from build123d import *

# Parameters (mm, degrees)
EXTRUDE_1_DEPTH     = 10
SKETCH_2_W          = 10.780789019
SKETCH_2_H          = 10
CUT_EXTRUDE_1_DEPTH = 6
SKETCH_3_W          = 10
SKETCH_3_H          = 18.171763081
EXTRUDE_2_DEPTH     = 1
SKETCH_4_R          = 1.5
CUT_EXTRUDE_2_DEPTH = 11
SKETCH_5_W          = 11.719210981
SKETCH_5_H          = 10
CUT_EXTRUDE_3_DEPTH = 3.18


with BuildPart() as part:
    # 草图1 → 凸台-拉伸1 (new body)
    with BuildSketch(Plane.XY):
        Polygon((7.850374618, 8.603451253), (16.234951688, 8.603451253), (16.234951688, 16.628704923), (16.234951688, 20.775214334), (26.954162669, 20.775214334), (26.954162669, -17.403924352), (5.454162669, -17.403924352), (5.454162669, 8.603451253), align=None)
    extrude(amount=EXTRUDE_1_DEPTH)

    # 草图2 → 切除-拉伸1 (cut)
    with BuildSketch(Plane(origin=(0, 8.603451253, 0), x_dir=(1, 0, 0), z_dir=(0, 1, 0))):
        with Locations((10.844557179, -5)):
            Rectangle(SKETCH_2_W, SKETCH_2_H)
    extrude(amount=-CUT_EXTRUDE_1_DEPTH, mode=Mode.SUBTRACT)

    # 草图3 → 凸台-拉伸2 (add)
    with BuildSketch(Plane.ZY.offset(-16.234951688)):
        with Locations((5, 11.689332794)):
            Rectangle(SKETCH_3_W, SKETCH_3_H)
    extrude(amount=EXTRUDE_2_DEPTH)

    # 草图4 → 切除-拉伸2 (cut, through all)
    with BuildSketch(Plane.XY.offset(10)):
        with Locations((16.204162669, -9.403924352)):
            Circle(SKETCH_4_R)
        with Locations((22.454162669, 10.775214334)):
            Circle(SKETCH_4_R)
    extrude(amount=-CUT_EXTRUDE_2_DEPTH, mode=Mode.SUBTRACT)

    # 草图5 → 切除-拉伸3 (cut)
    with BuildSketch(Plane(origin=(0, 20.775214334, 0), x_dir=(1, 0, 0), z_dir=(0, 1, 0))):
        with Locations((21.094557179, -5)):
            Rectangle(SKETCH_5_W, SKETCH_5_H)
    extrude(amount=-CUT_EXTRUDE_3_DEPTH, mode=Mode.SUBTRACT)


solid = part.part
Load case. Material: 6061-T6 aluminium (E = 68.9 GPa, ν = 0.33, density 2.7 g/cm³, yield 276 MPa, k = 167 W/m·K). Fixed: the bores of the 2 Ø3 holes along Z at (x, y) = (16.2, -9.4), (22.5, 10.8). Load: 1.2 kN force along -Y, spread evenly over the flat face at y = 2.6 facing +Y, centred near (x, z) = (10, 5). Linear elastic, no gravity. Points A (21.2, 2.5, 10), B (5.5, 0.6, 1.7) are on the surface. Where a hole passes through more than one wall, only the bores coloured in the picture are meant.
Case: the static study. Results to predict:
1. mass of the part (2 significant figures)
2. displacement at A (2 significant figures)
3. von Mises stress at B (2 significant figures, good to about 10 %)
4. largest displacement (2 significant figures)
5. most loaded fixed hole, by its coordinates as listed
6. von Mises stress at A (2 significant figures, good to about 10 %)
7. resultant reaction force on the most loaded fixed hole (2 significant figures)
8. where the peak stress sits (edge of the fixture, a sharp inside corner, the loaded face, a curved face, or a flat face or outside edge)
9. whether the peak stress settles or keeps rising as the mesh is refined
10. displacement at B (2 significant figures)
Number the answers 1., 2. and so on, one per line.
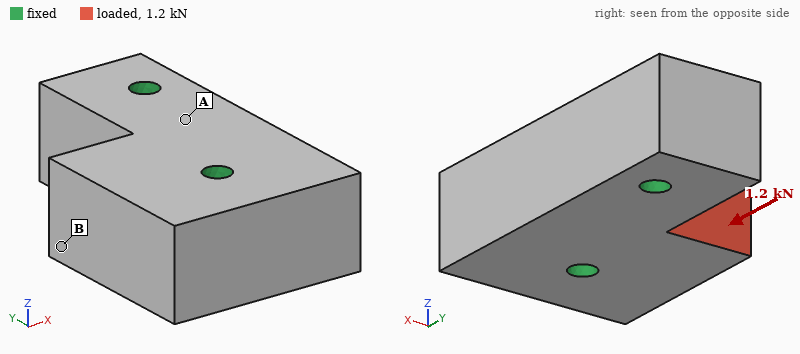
1. 16 g
2. 0.96 µm
3. 13 MPa
4. 5.5 µm
5. (16.2, -9.4)
6. 4.3 MPa
7. 1.1 kN
8. edge of the fixture
9. keeps rising
10. 4.9 µm
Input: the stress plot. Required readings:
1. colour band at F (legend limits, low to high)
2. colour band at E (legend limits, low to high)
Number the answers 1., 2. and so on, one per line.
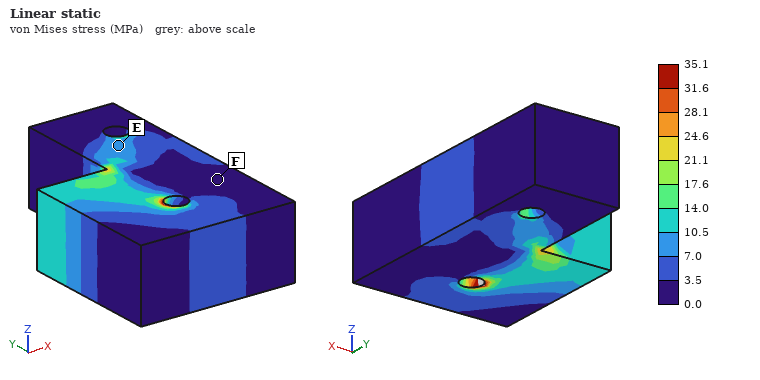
1. 0.0 to 3.5 MPa
2. 7.0 to 10.5 MPa
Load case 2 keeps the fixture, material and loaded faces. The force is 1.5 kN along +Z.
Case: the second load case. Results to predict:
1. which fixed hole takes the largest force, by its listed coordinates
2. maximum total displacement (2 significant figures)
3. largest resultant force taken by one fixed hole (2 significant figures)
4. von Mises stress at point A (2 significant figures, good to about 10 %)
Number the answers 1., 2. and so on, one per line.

1. (16.2, -9.4)
2. 25 µm
3. 970 N
4. 18 MPa
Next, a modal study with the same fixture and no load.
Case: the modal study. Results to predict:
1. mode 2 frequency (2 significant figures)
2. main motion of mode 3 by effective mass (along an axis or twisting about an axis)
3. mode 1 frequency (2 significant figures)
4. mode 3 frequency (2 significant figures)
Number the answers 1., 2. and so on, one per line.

1. 35 kHz
2. along Z
3. 33 kHz
4. 43 kHz
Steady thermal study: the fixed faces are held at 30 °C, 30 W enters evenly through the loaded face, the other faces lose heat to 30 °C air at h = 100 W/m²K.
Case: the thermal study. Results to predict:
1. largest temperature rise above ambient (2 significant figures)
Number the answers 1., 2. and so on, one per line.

1. 18 K
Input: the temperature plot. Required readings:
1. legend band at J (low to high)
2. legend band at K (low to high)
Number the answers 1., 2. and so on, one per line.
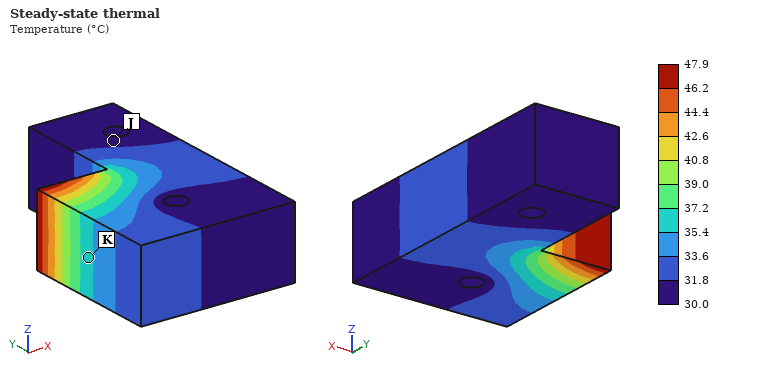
1. 30.0 to 31.8 °C
2. 35.4 to 37.2 °C
